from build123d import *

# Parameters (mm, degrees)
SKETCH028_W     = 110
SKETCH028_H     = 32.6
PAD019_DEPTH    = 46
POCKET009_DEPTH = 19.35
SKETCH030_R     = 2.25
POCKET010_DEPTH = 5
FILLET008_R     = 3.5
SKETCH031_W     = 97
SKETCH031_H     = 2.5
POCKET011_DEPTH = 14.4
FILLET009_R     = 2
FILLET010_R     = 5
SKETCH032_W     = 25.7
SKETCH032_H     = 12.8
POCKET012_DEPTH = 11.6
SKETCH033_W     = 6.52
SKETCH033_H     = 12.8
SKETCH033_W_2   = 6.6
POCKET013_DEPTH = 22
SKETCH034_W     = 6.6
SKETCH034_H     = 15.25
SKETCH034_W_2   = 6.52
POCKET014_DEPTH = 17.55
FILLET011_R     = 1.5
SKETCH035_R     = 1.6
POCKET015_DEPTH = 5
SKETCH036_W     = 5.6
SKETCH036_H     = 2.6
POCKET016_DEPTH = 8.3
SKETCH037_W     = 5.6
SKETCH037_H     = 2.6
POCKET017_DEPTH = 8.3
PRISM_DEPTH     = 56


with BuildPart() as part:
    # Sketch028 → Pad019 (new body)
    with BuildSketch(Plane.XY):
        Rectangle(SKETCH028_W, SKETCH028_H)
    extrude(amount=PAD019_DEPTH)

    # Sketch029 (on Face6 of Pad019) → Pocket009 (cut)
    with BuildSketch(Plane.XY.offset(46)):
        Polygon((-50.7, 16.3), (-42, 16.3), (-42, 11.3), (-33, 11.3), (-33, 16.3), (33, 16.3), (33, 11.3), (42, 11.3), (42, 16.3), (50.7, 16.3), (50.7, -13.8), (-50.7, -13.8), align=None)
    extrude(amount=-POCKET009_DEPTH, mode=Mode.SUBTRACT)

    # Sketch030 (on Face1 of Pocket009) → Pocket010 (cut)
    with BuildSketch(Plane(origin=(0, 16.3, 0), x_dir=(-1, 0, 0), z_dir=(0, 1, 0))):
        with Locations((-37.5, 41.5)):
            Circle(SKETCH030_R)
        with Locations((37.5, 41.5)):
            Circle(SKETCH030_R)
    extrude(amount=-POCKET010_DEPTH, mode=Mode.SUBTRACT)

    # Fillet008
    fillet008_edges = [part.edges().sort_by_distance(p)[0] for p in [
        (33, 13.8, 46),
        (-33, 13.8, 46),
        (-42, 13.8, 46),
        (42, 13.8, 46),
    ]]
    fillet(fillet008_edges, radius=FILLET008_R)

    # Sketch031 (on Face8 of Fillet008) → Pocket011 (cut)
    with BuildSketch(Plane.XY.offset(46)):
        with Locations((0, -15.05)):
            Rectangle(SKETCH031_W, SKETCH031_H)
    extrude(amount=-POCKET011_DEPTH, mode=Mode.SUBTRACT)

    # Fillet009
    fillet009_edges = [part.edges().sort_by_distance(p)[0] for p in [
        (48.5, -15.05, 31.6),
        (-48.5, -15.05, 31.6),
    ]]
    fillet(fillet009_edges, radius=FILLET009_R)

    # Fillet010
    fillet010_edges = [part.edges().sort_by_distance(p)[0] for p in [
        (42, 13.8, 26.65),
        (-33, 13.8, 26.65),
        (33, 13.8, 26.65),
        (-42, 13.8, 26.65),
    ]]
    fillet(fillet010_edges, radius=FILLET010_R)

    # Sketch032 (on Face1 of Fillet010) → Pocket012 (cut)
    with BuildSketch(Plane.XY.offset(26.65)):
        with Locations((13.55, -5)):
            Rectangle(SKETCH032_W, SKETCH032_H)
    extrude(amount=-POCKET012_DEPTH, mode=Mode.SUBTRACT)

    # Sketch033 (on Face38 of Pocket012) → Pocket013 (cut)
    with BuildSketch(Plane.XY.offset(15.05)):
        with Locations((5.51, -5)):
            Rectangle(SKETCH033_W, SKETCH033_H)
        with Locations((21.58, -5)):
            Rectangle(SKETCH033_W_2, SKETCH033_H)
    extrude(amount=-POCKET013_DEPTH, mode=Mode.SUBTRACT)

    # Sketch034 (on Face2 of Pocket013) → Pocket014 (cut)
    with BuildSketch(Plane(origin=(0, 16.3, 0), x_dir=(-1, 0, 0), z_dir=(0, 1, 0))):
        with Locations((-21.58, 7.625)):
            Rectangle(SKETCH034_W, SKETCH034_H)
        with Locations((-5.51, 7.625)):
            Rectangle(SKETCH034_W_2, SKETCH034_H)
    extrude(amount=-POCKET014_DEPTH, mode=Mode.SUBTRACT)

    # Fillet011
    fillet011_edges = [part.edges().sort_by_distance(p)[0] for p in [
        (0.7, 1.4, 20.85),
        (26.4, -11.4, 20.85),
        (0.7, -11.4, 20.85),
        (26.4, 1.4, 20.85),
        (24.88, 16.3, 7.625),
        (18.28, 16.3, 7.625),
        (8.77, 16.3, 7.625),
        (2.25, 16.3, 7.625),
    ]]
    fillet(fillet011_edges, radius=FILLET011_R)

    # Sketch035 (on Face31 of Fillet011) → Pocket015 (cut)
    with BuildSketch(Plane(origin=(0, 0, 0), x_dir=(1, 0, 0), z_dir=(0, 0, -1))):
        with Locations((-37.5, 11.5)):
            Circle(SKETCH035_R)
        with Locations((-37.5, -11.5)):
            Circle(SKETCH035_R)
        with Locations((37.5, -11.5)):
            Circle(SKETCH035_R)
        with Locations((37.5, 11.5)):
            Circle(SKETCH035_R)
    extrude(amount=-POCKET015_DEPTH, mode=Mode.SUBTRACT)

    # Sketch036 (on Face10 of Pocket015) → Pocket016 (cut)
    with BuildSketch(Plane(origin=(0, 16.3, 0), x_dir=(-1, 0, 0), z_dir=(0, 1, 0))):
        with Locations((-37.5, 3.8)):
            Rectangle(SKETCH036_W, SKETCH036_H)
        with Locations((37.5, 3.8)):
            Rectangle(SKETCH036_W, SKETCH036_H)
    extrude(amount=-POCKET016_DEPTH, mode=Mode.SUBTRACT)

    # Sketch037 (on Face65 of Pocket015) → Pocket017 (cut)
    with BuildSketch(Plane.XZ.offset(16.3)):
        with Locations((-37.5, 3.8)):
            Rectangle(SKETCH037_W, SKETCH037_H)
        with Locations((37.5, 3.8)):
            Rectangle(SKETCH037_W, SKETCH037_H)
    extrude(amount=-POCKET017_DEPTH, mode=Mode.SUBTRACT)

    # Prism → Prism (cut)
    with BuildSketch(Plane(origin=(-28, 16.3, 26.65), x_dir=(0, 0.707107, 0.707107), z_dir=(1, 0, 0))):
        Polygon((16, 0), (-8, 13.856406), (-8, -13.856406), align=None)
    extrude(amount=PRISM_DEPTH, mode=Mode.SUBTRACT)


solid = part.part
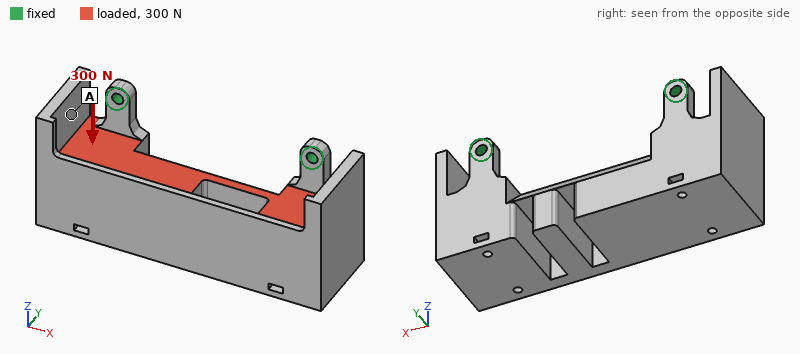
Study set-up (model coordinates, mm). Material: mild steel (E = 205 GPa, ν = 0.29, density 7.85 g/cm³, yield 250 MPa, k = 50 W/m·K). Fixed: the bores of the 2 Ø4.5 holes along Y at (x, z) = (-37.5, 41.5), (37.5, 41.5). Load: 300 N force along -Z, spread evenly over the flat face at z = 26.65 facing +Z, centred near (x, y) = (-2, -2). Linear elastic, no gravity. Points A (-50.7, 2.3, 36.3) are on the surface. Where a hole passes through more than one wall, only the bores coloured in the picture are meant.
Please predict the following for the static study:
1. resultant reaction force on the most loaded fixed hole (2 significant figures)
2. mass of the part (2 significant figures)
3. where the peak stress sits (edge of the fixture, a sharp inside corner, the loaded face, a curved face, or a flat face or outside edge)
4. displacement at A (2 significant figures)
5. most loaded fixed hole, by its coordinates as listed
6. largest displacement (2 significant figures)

160 N
710 g
a flat face or outside edge
21 µm
(-37.5, 41.5)
78 µm
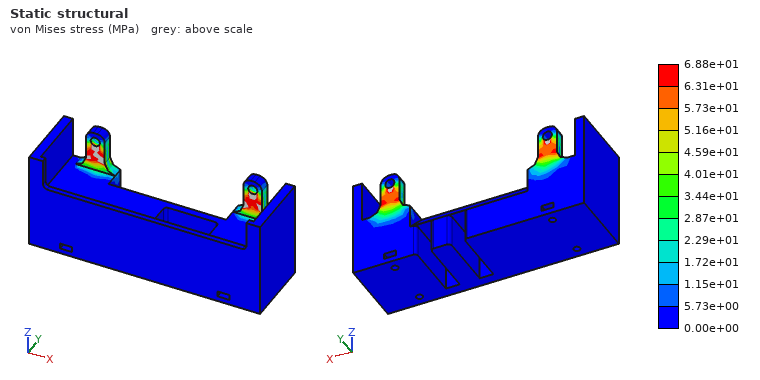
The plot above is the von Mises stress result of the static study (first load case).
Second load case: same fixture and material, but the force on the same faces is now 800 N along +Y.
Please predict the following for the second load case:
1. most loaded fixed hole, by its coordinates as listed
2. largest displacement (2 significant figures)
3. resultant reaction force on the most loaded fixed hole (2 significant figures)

(-37.5, 41.5)
87 µm
420 N
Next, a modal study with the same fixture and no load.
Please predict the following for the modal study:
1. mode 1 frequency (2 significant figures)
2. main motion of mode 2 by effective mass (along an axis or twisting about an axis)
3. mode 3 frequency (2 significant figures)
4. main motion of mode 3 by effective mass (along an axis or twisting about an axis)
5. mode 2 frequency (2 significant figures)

370 Hz
along X
2400 Hz
along X
1700 Hz
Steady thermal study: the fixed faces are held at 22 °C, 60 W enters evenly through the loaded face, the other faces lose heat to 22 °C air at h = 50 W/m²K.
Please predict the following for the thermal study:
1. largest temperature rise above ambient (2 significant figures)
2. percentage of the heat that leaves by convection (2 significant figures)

58 K
77 %
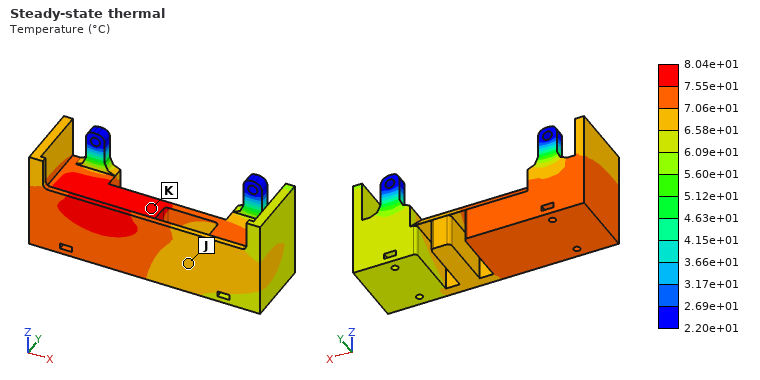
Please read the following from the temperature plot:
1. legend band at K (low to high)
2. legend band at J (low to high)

7.55e+01 to 8.04e+01 °C
6.58e+01 to 7.06e+01 °C
